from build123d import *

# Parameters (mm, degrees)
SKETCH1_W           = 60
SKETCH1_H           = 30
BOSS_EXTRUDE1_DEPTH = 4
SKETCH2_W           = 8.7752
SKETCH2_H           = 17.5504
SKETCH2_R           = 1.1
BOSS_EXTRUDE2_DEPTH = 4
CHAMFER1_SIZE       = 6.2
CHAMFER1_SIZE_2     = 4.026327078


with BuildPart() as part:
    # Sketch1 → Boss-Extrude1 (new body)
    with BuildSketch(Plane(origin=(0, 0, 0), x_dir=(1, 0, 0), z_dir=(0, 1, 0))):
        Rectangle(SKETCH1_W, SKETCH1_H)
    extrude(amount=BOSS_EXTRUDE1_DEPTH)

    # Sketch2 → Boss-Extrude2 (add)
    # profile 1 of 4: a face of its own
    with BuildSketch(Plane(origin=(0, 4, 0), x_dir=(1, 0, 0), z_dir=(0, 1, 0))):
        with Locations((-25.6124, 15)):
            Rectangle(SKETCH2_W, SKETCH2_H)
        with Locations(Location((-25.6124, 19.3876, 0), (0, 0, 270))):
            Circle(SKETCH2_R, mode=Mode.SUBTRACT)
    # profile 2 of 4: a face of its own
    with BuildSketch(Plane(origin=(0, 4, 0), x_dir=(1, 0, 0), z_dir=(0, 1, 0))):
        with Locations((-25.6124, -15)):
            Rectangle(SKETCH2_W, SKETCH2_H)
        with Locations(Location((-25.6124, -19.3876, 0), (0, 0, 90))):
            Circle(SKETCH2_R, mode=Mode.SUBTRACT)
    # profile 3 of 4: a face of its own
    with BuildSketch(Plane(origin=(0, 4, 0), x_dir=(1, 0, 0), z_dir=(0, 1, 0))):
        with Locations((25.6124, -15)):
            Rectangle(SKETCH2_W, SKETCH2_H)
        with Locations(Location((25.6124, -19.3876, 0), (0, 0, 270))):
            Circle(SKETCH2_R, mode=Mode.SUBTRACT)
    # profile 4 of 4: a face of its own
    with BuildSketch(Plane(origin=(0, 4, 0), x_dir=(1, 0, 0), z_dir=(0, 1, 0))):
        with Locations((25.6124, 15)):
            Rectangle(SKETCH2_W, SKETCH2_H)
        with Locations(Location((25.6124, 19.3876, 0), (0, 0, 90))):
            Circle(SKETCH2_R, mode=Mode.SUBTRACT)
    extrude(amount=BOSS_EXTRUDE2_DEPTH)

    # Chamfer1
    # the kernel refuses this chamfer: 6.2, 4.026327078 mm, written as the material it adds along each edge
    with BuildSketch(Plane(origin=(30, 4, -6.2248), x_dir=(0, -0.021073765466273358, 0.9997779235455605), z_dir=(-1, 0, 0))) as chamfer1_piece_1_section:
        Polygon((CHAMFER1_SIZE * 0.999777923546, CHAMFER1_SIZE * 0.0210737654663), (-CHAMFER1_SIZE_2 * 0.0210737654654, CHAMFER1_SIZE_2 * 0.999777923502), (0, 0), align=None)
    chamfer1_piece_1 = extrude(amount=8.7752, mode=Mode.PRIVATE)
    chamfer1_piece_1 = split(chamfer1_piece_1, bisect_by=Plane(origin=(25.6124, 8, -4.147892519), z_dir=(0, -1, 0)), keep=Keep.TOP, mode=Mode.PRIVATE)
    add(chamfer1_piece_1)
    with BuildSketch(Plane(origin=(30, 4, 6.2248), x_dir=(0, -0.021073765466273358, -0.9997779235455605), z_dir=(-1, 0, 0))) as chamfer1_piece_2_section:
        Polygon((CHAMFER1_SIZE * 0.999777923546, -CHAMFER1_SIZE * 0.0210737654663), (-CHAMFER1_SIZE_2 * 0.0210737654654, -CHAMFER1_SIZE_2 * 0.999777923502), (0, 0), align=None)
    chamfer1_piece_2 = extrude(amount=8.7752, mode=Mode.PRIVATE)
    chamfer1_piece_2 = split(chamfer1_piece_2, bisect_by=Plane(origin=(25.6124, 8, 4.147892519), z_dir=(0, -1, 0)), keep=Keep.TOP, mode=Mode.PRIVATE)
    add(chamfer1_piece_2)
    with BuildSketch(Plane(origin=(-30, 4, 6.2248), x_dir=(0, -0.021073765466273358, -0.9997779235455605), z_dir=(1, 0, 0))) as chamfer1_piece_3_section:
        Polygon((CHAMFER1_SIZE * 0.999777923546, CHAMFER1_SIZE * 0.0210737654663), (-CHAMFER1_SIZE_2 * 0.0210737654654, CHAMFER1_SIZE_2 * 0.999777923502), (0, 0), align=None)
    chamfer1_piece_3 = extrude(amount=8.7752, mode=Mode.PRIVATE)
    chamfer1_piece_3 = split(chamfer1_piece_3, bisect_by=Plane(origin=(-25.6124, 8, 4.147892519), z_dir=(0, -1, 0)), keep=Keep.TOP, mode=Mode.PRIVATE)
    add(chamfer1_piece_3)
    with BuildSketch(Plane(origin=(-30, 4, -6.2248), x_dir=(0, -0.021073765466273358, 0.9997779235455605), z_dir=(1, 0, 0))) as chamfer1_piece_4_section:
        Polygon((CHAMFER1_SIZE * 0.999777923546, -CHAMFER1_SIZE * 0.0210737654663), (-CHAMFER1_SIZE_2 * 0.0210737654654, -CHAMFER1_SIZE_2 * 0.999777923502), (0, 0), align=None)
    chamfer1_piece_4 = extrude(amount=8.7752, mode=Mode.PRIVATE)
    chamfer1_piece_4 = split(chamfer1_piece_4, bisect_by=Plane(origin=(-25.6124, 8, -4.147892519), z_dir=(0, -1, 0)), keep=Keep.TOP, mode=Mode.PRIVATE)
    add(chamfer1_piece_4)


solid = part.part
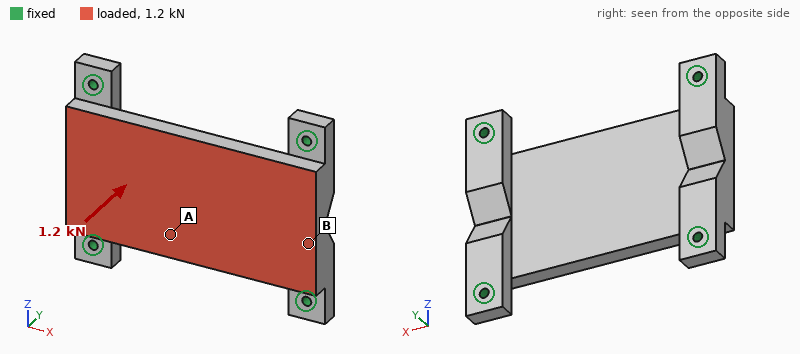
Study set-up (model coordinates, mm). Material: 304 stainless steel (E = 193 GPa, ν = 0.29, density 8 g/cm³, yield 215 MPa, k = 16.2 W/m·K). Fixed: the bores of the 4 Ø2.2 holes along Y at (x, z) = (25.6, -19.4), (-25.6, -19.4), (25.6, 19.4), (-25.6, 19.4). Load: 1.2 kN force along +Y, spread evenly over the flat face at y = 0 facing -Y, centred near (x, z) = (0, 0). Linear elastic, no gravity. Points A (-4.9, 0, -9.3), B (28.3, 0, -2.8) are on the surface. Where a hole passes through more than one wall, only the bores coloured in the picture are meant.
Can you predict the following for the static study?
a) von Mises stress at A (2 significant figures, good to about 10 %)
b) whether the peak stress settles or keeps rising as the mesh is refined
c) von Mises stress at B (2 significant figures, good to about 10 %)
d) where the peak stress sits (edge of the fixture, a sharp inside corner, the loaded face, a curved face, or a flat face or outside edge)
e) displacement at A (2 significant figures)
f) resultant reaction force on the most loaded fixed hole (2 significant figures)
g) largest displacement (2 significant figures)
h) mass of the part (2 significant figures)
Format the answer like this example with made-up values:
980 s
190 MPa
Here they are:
30 MPa
keeps rising
13 MPa
edge of the fixture
17 µm
560 N
18 µm
80 g
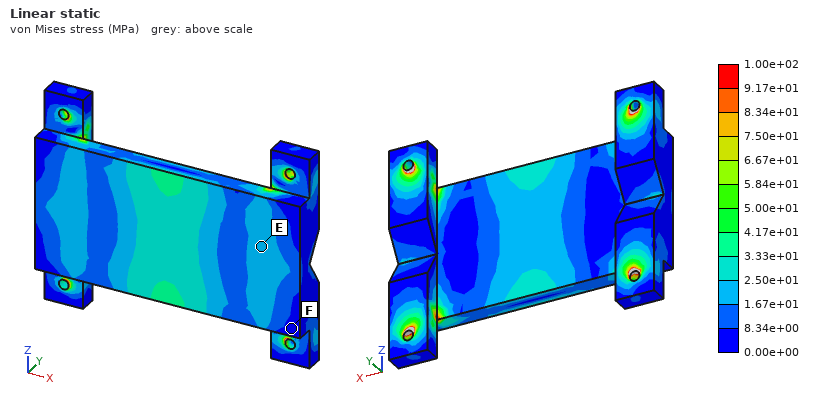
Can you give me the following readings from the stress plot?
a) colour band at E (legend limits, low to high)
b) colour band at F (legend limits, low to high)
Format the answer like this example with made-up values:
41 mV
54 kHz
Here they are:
1.67e+01 to 2.50e+01 MPa
0.00e+00 to 8.34e+00 MPa
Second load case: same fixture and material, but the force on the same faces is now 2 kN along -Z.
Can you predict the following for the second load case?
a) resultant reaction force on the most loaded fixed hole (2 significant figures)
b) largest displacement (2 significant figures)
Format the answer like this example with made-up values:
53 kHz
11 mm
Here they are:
550 N
4.4 µm
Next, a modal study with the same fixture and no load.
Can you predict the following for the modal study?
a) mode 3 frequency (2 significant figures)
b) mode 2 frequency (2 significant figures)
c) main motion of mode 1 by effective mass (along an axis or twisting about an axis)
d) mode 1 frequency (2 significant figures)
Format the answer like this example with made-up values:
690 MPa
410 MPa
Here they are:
11 kHz
11 kHz
along Y
6200 Hz
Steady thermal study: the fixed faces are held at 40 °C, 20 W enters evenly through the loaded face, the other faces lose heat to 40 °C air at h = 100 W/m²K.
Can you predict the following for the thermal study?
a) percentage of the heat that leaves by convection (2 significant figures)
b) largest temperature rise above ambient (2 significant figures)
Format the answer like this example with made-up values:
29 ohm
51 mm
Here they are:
59 %
55 K
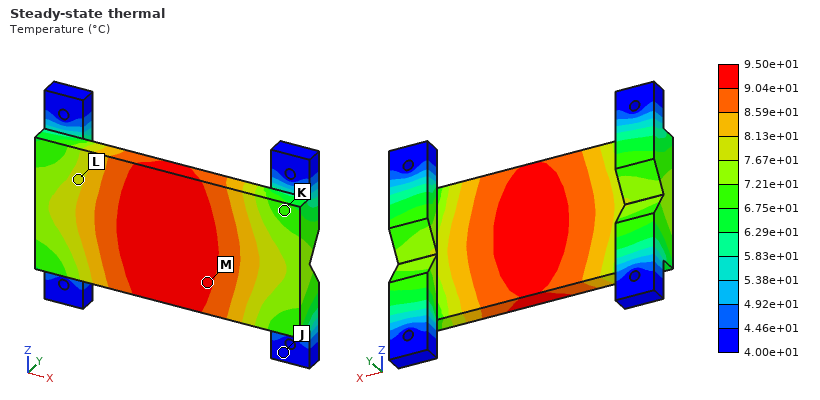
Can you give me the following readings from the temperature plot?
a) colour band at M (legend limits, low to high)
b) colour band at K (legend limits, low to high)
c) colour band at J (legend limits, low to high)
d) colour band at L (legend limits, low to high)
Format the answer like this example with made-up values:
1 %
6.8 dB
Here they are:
9.04e+01 to 9.50e+01 °C
6.75e+01 to 7.21e+01 °C
4.00e+01 to 4.46e+01 °C
7.67e+01 to 8.13e+01 °C
